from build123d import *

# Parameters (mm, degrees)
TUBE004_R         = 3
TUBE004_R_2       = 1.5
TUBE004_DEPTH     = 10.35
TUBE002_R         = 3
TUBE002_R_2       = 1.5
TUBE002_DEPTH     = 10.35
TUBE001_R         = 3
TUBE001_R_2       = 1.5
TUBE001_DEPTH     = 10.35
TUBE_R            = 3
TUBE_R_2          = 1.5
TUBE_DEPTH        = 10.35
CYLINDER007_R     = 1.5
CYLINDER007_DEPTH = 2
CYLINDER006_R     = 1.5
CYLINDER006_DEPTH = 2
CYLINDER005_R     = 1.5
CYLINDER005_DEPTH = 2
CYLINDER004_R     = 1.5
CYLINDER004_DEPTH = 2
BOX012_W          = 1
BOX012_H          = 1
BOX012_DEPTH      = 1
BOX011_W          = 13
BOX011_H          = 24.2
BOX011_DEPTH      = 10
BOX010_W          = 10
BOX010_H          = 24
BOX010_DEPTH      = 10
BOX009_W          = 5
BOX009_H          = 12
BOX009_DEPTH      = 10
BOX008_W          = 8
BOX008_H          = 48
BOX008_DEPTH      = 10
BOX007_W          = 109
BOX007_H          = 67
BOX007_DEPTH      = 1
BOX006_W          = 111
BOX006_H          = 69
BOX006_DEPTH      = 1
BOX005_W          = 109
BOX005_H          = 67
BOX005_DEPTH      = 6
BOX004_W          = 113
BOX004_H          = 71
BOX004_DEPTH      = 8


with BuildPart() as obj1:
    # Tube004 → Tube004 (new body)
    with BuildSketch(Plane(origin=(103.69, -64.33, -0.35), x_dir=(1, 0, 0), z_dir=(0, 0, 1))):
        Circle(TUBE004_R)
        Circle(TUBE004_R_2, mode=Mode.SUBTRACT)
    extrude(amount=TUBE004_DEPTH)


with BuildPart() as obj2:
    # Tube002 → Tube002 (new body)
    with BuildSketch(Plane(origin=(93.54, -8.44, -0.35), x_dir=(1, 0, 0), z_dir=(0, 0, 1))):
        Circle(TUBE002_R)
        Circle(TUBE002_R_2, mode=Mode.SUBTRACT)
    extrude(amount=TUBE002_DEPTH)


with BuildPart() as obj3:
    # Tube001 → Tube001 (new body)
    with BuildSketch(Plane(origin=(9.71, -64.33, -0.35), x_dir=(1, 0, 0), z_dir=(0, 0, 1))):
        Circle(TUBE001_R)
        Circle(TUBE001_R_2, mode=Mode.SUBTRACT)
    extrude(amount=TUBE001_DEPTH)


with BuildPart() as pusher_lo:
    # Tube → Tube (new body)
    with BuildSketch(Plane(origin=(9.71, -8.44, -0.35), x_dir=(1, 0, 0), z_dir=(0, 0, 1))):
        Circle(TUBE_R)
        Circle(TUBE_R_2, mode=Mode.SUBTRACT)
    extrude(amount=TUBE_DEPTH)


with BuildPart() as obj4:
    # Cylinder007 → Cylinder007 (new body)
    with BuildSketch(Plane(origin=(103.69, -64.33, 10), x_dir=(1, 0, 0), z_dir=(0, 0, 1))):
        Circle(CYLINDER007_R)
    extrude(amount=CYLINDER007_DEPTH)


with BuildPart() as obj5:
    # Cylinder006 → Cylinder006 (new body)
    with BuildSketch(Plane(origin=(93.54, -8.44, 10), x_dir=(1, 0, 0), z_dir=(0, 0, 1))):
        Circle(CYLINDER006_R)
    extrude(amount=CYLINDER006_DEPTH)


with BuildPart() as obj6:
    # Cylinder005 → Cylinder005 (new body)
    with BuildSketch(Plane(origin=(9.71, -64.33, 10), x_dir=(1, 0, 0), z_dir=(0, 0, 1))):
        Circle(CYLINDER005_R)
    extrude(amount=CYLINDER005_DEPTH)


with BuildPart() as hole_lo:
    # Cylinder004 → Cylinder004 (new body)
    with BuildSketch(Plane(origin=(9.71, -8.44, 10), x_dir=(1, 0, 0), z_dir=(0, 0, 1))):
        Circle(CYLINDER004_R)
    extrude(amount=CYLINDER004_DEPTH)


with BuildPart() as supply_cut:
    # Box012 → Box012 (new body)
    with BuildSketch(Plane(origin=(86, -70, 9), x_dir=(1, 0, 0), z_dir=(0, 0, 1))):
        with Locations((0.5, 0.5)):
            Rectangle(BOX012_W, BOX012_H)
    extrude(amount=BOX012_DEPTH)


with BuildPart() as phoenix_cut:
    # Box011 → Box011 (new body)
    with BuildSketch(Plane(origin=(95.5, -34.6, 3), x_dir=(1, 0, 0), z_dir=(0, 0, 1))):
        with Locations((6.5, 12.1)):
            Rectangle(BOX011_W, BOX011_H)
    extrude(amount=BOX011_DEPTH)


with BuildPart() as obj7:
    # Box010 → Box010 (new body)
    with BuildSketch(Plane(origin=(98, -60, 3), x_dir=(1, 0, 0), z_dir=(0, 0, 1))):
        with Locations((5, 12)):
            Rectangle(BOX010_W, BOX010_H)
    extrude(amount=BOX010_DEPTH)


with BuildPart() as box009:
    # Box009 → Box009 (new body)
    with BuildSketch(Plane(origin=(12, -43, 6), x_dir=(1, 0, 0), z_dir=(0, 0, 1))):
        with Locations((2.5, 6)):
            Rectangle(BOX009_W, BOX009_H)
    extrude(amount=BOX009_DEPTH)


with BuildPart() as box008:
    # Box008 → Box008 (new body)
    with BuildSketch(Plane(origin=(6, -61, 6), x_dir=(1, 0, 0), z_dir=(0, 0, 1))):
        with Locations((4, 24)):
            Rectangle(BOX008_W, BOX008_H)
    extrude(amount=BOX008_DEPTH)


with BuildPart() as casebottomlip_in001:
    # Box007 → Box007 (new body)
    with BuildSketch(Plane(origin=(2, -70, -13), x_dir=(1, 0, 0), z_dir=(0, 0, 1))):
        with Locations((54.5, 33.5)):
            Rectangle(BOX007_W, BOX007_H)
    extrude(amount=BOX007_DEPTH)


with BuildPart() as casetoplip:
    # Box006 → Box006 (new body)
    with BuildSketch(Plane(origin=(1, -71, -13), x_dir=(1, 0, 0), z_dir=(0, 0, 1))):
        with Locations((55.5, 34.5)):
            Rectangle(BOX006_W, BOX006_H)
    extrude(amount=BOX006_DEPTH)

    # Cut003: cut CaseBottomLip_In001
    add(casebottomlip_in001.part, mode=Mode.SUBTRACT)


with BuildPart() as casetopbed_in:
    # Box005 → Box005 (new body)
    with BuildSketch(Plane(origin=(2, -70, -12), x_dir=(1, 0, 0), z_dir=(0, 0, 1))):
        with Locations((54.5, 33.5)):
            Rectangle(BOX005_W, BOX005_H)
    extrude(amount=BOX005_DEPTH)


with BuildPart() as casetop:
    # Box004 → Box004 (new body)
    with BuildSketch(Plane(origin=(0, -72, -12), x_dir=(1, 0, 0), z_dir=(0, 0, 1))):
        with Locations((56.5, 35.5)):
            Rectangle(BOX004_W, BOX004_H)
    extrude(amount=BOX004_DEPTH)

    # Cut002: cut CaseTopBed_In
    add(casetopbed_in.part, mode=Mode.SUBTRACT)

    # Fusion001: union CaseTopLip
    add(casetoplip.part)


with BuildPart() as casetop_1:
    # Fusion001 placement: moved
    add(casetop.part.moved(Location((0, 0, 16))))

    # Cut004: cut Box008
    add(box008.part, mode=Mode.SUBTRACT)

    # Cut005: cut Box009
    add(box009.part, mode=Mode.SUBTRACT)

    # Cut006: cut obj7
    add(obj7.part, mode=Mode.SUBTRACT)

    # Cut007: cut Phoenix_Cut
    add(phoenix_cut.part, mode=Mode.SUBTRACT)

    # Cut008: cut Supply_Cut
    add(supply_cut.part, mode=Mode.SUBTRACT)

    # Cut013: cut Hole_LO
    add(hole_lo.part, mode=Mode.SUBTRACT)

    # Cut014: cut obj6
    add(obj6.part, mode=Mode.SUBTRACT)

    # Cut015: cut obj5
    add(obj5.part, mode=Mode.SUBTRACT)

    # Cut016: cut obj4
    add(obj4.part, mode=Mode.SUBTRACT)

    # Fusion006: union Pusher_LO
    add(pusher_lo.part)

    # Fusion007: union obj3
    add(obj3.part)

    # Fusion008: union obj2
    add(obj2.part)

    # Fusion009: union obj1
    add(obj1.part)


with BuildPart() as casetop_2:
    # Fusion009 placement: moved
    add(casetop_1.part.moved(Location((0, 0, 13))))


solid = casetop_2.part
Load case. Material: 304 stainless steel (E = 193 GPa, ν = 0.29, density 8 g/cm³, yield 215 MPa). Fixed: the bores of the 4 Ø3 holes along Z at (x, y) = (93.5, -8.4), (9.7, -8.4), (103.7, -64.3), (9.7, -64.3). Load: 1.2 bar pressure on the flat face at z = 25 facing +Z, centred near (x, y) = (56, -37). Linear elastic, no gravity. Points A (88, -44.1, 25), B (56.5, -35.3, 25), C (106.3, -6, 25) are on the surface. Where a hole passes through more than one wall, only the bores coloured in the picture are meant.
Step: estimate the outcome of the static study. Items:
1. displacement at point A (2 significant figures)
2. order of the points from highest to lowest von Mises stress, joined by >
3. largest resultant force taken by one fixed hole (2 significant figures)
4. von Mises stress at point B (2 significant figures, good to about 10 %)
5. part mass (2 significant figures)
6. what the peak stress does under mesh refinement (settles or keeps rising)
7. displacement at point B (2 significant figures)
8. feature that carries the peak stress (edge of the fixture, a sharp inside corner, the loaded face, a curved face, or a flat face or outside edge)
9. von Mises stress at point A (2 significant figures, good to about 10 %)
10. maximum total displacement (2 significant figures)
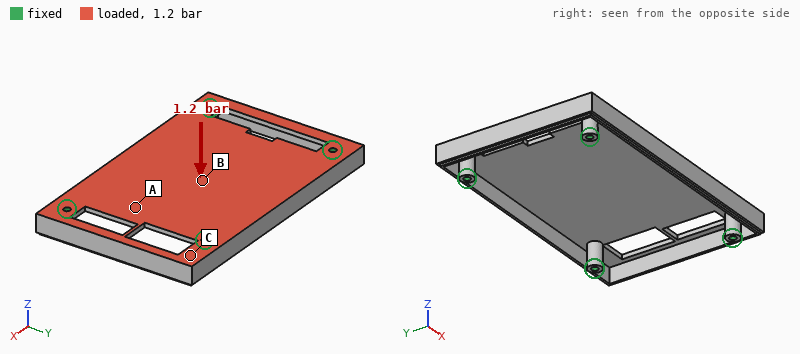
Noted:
0.062 mm
B > A > C
250 N
47 MPa
160 g
keeps rising
0.12 mm
edge of the fixture
32 MPa
0.12 mm
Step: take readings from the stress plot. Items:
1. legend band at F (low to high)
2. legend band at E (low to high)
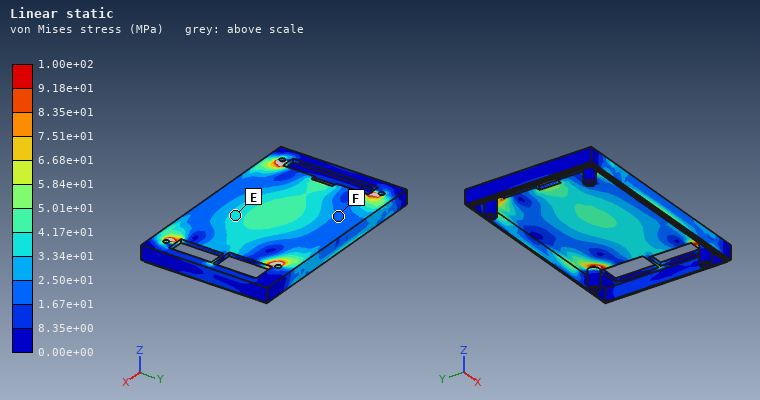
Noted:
1.67e+01 to 2.50e+01 MPa
3.34e+01 to 4.17e+01 MPa
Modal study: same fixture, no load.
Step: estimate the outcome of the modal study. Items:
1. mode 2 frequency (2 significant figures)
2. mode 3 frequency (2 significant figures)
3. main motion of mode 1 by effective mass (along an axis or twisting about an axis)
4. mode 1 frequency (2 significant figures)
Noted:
2700 Hz
3000 Hz
along Z
1500 Hz
